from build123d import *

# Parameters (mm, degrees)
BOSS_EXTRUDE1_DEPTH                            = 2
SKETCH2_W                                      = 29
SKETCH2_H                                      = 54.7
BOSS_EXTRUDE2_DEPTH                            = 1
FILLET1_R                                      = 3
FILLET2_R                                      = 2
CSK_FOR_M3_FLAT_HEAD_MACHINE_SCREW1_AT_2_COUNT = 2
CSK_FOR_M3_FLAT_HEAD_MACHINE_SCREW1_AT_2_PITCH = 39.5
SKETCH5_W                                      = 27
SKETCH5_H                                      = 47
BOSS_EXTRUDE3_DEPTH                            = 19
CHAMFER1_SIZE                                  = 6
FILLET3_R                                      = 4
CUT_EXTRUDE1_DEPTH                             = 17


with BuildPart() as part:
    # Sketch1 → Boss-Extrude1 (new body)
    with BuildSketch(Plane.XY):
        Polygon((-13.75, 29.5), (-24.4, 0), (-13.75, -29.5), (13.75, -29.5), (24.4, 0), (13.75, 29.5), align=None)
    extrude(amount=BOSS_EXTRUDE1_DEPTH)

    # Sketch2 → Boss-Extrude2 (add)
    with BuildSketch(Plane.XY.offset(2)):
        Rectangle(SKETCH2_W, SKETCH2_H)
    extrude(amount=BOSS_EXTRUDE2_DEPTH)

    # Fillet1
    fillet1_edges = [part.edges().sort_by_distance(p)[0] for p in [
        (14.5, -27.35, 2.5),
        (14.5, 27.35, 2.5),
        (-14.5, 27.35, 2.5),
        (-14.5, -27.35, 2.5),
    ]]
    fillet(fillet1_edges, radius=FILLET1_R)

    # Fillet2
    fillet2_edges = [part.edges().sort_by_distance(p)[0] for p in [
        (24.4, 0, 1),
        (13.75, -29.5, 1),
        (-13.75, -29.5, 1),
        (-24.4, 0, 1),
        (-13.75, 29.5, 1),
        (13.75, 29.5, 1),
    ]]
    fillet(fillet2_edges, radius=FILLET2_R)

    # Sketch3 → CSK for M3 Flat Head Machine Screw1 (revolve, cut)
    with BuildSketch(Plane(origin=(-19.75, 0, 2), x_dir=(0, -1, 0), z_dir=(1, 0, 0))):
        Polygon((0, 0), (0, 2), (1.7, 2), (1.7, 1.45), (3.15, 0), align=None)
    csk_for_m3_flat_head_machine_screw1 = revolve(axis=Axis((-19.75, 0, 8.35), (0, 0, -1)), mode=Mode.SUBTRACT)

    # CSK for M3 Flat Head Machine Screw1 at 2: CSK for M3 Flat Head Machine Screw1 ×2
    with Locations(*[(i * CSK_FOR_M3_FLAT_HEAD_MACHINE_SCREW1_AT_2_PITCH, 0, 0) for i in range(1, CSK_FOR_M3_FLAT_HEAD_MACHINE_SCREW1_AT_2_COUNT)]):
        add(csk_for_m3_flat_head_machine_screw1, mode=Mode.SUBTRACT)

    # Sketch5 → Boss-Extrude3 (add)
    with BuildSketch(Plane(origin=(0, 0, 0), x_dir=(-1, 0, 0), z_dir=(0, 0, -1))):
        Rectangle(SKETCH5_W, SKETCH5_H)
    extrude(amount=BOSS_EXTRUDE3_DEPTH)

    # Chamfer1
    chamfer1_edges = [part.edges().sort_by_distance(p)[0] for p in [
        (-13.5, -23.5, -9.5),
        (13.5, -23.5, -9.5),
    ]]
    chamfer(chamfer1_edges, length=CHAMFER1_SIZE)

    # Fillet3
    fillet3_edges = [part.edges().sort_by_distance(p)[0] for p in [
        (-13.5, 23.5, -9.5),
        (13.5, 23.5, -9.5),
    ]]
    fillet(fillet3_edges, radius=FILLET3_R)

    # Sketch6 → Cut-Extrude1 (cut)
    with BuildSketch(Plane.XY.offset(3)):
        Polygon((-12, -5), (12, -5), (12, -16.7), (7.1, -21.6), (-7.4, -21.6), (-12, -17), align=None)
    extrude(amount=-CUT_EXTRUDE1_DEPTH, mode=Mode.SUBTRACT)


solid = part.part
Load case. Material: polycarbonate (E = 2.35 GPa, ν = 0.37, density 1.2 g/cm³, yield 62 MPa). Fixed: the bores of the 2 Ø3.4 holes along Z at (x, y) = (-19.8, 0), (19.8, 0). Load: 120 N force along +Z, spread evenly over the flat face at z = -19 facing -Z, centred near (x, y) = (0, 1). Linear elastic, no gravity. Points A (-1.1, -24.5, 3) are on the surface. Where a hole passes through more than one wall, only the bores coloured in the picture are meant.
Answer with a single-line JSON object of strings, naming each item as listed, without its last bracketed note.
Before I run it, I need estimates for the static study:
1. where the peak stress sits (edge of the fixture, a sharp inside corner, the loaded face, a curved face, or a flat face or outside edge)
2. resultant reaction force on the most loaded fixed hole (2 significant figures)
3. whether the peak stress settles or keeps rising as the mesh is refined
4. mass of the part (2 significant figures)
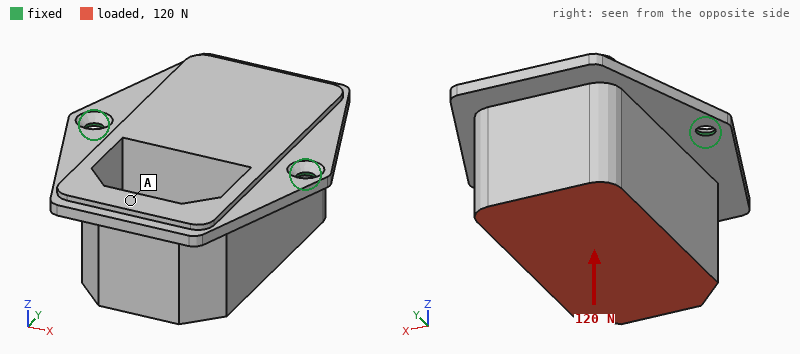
{"where the peak stress sits": "edge of the fixture", "resultant reaction force on the most loaded fixed hole": "71 N", "whether the peak stress settles or keeps rising as the mesh is refined": "keeps rising", "mass of the part": "28 g"}
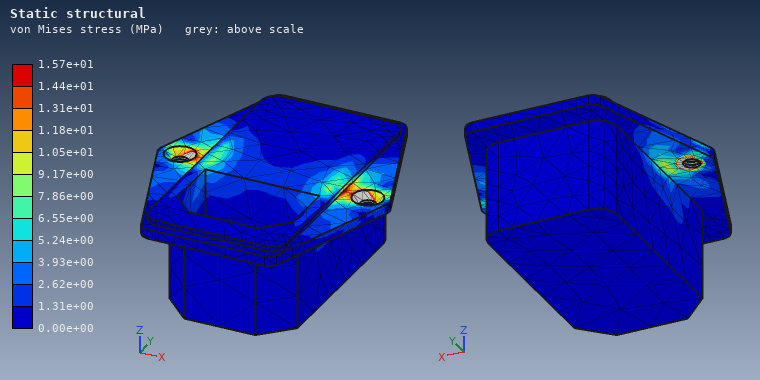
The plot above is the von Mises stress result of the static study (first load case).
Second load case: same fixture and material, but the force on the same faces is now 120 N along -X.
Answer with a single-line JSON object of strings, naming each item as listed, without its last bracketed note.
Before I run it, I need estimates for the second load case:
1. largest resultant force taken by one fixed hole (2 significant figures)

{"largest resultant force taken by one fixed hole": "89 N"}
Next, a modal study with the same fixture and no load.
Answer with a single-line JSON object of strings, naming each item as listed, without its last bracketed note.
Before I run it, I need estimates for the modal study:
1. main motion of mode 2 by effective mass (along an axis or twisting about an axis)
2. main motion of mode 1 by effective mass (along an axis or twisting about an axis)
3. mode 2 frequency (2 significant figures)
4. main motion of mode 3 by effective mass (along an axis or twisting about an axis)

{"main motion of mode 2 by effective mass": "along Z", "main motion of mode 1 by effective mass": "along Y", "mode 2 frequency": "970 Hz", "main motion of mode 3 by effective mass": "along X"}
